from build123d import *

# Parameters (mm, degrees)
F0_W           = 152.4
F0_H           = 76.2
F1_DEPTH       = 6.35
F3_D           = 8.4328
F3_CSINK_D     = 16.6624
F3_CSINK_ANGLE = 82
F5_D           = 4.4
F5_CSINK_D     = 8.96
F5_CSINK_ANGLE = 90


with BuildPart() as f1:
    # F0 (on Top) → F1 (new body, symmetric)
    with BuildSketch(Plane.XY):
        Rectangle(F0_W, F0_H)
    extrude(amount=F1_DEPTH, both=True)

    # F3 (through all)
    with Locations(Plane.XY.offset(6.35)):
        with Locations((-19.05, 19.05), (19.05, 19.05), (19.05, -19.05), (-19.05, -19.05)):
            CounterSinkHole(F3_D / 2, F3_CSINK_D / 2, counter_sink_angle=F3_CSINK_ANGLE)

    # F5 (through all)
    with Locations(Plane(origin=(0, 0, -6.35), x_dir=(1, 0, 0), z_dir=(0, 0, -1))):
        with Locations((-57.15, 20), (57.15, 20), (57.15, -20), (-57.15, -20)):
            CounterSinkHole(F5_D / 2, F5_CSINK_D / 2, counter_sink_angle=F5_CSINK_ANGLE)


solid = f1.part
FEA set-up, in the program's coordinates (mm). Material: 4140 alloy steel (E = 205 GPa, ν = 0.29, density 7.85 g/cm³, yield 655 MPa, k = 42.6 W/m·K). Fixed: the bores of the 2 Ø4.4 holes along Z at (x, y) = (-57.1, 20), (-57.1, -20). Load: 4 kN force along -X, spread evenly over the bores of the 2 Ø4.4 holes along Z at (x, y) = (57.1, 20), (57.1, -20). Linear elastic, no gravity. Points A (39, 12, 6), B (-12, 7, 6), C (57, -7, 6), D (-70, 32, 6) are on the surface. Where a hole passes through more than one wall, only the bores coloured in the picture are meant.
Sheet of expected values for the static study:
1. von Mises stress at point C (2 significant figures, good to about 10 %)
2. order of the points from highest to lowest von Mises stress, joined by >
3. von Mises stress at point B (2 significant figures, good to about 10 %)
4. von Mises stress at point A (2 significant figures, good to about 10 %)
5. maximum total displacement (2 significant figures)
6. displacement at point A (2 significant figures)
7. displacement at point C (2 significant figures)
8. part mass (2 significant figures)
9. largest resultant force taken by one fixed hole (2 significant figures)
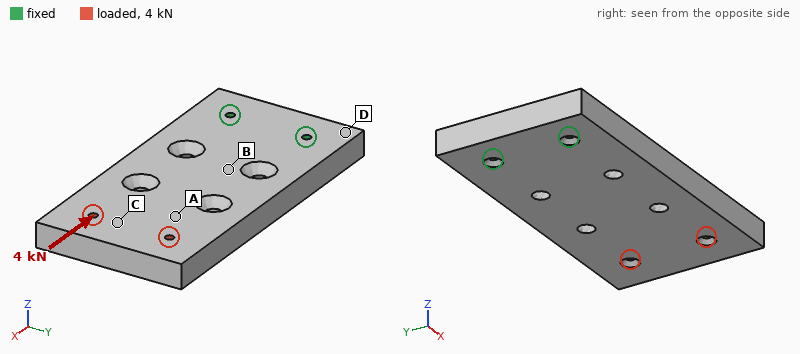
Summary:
3.5 MPa
B > A > C > D
8.5 MPa
6.7 MPa
19 µm
10 µm
14 µm
1.1 kg
2.0 kN
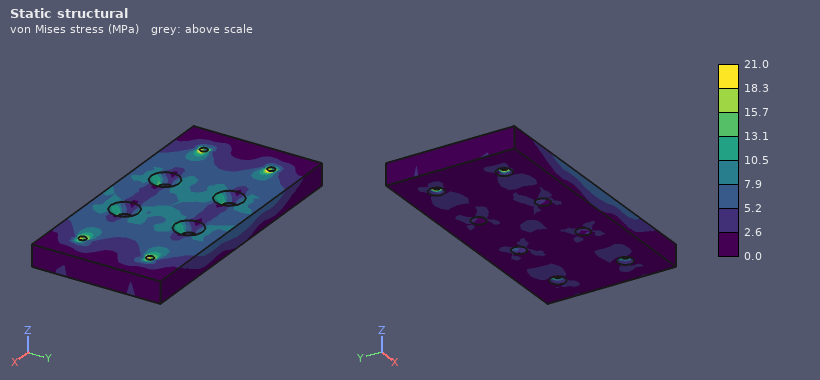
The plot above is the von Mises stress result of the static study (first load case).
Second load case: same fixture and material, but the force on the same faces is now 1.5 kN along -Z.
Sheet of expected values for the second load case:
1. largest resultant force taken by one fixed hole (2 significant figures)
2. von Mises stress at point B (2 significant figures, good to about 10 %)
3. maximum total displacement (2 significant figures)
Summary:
770 N
64 MPa
0.47 mm
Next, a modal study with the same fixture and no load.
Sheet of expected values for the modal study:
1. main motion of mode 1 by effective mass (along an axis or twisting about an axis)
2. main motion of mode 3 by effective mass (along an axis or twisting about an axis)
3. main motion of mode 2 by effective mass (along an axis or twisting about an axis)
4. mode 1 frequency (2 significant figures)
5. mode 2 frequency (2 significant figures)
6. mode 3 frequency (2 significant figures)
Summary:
along Z
along Y
twisting about X
510 Hz
1900 Hz
2300 Hz
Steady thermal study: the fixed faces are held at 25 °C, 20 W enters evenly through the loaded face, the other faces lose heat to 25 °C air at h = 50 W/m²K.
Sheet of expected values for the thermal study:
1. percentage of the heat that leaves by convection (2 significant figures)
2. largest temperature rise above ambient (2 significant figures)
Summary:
78 %
29 K
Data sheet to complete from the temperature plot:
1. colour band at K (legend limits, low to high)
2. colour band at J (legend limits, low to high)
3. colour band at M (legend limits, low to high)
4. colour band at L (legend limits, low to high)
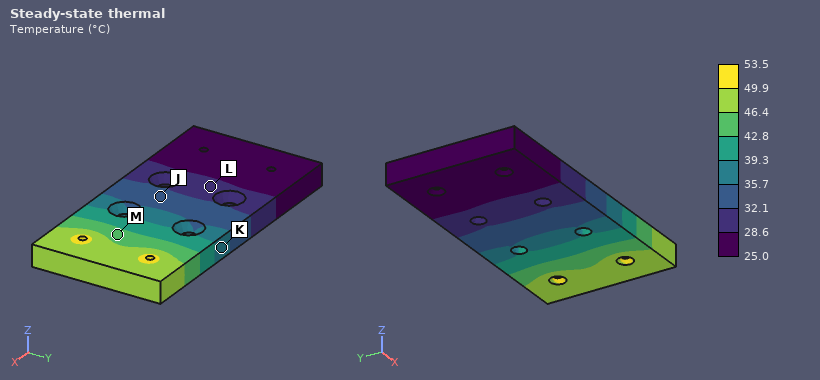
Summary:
35.7 to 39.3 °C
32.1 to 35.7 °C
42.8 to 46.4 °C
28.6 to 32.1 °C
